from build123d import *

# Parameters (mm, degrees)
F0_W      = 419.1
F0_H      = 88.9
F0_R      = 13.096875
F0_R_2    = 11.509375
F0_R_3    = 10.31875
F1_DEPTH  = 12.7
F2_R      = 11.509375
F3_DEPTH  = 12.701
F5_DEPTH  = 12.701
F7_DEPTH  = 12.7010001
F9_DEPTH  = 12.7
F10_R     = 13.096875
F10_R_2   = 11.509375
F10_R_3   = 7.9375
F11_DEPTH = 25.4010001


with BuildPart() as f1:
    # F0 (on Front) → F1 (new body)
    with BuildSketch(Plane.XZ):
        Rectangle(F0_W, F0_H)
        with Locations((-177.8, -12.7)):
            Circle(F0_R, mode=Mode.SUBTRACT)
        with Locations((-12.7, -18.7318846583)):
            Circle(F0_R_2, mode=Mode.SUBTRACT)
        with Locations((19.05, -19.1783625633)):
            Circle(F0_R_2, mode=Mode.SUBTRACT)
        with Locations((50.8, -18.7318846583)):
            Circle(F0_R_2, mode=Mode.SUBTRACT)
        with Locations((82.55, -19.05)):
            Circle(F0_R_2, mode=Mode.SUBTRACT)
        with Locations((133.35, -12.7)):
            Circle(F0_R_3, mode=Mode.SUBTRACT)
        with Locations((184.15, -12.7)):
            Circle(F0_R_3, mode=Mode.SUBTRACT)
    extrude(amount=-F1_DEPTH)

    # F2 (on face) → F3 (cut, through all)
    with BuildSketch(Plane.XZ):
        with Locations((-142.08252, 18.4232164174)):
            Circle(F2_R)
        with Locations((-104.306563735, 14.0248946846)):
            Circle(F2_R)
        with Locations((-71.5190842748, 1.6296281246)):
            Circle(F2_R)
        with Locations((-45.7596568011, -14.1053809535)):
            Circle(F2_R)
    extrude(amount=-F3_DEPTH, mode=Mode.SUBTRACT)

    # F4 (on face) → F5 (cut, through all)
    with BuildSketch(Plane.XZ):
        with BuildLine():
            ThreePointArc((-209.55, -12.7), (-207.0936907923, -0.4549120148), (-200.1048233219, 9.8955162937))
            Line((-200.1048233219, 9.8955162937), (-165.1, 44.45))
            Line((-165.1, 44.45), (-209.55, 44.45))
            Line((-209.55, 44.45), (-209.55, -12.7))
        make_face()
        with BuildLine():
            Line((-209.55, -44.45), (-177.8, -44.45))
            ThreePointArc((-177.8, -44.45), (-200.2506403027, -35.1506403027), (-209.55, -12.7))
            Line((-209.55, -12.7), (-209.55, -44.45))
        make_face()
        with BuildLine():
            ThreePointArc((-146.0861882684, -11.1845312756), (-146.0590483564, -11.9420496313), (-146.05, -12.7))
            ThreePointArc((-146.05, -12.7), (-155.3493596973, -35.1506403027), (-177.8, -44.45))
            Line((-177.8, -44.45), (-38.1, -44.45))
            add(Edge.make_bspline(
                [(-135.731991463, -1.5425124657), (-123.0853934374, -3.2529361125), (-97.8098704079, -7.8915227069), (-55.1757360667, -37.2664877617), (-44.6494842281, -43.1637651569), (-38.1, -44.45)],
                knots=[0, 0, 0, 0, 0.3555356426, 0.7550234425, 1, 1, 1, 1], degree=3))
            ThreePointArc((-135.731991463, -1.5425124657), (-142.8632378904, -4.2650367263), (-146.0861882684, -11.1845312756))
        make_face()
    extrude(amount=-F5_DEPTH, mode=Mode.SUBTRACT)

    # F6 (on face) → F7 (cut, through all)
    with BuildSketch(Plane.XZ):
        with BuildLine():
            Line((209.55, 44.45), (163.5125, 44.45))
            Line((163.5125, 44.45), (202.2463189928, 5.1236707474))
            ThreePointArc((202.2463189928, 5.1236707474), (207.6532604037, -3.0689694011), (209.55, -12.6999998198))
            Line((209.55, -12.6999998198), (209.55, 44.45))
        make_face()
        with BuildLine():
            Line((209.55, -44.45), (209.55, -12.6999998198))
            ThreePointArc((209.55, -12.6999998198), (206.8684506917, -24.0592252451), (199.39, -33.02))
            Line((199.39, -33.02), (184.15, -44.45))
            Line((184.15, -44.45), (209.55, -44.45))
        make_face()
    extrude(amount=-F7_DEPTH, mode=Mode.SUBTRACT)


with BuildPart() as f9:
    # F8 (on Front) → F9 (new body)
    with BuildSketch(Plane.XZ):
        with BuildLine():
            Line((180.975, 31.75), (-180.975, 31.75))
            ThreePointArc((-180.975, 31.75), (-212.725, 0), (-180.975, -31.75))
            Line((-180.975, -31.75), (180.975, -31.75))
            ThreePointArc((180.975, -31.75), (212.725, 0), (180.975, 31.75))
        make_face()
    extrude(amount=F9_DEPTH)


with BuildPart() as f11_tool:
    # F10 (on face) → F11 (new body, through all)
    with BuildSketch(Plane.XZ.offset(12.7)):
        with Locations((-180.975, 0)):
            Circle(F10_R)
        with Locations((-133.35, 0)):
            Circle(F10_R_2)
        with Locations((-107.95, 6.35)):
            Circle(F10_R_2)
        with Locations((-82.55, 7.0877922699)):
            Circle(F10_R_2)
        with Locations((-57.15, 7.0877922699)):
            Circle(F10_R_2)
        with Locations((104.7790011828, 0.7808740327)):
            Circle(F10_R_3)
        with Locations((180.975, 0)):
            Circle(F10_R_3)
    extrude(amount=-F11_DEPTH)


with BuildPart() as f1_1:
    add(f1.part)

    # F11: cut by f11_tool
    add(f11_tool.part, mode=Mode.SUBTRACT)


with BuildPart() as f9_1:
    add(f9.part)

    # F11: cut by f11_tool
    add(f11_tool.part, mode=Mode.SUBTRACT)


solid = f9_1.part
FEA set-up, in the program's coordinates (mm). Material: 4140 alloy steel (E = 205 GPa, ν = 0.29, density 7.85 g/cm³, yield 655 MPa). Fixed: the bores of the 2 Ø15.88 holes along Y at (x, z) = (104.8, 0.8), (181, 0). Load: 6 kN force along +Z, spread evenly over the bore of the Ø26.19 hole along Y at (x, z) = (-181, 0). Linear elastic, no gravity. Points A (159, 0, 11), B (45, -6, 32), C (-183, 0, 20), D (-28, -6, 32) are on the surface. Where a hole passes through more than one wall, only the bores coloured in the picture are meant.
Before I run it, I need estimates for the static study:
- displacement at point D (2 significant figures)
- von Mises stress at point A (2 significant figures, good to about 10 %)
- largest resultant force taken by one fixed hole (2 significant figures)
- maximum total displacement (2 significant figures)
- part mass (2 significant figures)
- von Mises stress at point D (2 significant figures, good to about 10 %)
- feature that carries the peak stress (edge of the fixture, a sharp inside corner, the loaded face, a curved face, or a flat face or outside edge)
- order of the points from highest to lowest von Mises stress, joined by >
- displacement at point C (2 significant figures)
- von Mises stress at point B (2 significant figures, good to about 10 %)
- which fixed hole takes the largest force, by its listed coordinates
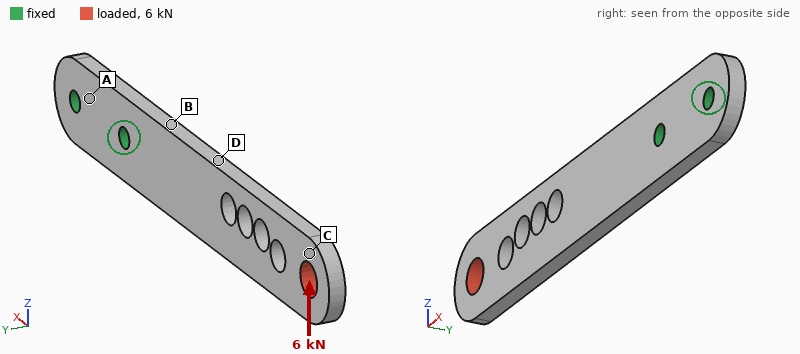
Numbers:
0.36 mm
42 MPa
20 kN
1.3 mm
2.3 kg
110 MPa
edge of the fixture
B > D > A > C
1.2 mm
160 MPa
(104.8, 0.8)
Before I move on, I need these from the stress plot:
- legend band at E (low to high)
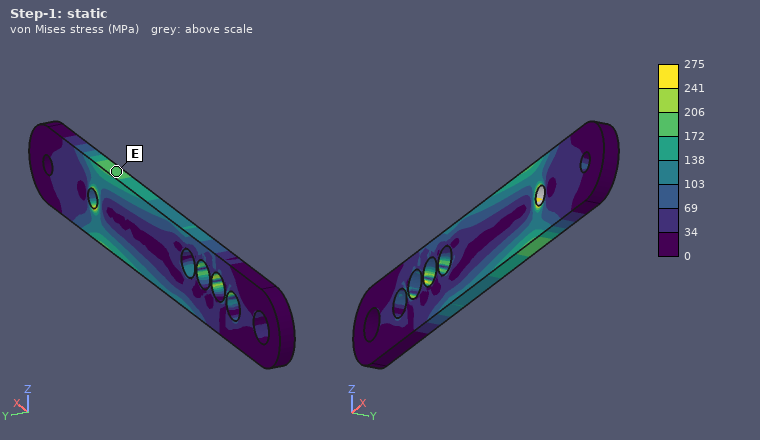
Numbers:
172 to 206 MPa
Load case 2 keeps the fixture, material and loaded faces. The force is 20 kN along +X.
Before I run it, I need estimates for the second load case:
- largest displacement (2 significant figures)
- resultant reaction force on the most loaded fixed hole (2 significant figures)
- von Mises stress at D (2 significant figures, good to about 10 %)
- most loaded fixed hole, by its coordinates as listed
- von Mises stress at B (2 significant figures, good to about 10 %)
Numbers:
49 µm
18 kN
36 MPa
(104.8, 0.8)
25 MPa
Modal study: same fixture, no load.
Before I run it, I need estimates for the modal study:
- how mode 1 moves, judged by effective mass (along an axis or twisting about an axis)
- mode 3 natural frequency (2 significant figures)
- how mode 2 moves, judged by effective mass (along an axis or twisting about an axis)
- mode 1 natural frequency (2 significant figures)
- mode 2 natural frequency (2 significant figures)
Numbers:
along Y
660 Hz
along Z
120 Hz
500 Hz
